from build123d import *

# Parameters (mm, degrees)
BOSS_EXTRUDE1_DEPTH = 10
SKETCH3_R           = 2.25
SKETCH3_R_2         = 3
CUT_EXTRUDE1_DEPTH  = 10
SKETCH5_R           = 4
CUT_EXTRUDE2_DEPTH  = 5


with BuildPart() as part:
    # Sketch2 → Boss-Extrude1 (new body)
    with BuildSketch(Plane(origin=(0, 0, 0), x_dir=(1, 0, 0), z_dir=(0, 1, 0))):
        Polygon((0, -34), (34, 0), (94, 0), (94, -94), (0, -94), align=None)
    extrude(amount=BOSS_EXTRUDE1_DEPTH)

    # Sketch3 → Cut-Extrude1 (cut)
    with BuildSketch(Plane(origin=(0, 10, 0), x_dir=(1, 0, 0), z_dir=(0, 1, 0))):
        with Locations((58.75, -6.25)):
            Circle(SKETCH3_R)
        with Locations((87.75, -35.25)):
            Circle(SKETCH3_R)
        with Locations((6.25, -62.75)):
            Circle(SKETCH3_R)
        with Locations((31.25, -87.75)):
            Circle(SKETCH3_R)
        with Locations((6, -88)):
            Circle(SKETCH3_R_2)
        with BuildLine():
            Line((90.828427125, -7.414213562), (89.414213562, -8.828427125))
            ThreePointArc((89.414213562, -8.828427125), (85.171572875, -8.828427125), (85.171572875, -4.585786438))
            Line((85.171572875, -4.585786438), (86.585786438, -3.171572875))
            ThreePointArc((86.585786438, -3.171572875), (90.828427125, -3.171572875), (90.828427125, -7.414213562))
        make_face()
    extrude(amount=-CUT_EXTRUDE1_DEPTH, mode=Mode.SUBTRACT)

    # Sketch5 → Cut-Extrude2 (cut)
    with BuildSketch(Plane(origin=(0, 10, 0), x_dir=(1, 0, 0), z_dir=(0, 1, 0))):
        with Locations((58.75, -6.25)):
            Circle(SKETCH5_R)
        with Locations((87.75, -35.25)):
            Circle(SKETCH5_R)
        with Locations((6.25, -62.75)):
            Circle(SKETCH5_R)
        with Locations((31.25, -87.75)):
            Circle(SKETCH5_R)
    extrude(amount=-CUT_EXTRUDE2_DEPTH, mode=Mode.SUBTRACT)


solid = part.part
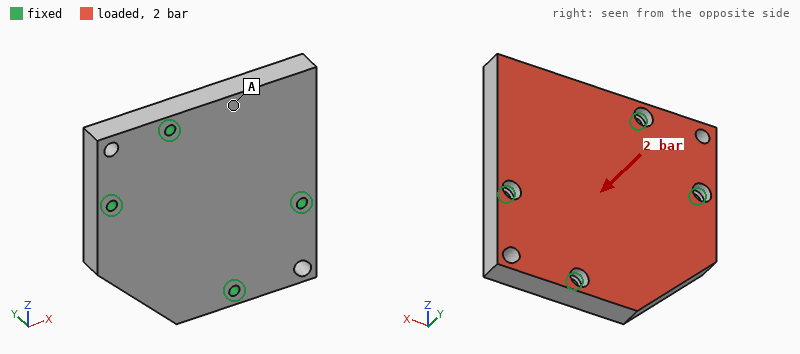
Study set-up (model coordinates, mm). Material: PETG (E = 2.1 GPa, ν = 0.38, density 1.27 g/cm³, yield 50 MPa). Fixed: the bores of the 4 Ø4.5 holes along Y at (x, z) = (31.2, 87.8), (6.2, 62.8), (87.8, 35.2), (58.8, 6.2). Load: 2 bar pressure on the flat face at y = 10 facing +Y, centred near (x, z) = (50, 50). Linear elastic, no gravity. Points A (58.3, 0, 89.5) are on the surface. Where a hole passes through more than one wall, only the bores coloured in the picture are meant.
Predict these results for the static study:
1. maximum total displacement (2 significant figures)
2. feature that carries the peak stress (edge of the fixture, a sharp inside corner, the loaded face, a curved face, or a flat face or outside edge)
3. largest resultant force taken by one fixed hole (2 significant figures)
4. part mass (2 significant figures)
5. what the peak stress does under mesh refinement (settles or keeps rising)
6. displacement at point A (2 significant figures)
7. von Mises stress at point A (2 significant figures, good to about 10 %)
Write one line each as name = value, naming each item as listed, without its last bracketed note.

maximum total displacement = 0.99 mm
feature that carries the peak stress = edge of the fixture
largest resultant force taken by one fixed hole = 580 N
part mass = 100 g
what the peak stress does under mesh refinement = keeps rising
displacement at point A = 0.44 mm
von Mises stress at point A = 4.3 MPa
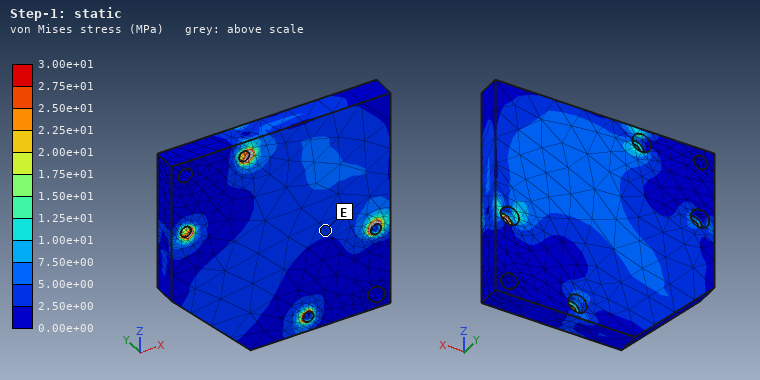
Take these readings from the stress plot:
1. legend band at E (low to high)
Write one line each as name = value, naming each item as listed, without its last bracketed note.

legend band at E = 2.50e+00 to 5.00e+00 MPa
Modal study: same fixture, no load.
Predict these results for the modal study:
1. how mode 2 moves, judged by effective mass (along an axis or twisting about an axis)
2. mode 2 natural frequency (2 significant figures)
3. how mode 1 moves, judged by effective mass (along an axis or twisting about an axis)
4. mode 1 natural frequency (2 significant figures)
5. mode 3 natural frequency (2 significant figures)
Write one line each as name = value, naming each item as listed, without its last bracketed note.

how mode 2 moves, judged by effective mass = along Y
mode 2 natural frequency = 1300 Hz
how mode 1 moves, judged by effective mass = along Y
mode 1 natural frequency = 870 Hz
mode 3 natural frequency = 2100 Hz
